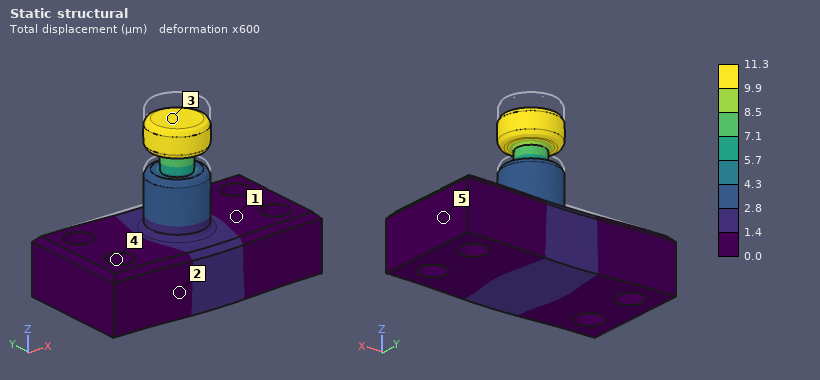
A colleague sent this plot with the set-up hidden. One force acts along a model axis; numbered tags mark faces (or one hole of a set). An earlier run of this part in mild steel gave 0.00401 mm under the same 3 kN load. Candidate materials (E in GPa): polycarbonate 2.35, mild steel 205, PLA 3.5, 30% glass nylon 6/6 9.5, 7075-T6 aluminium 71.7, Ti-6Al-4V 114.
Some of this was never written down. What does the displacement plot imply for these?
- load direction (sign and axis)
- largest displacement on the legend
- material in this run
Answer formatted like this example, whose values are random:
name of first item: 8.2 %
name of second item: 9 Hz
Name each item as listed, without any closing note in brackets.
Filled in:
load direction: -Z
largest displacement on the legend: 11.3 µm
material in this run: 7075-T6 aluminium
